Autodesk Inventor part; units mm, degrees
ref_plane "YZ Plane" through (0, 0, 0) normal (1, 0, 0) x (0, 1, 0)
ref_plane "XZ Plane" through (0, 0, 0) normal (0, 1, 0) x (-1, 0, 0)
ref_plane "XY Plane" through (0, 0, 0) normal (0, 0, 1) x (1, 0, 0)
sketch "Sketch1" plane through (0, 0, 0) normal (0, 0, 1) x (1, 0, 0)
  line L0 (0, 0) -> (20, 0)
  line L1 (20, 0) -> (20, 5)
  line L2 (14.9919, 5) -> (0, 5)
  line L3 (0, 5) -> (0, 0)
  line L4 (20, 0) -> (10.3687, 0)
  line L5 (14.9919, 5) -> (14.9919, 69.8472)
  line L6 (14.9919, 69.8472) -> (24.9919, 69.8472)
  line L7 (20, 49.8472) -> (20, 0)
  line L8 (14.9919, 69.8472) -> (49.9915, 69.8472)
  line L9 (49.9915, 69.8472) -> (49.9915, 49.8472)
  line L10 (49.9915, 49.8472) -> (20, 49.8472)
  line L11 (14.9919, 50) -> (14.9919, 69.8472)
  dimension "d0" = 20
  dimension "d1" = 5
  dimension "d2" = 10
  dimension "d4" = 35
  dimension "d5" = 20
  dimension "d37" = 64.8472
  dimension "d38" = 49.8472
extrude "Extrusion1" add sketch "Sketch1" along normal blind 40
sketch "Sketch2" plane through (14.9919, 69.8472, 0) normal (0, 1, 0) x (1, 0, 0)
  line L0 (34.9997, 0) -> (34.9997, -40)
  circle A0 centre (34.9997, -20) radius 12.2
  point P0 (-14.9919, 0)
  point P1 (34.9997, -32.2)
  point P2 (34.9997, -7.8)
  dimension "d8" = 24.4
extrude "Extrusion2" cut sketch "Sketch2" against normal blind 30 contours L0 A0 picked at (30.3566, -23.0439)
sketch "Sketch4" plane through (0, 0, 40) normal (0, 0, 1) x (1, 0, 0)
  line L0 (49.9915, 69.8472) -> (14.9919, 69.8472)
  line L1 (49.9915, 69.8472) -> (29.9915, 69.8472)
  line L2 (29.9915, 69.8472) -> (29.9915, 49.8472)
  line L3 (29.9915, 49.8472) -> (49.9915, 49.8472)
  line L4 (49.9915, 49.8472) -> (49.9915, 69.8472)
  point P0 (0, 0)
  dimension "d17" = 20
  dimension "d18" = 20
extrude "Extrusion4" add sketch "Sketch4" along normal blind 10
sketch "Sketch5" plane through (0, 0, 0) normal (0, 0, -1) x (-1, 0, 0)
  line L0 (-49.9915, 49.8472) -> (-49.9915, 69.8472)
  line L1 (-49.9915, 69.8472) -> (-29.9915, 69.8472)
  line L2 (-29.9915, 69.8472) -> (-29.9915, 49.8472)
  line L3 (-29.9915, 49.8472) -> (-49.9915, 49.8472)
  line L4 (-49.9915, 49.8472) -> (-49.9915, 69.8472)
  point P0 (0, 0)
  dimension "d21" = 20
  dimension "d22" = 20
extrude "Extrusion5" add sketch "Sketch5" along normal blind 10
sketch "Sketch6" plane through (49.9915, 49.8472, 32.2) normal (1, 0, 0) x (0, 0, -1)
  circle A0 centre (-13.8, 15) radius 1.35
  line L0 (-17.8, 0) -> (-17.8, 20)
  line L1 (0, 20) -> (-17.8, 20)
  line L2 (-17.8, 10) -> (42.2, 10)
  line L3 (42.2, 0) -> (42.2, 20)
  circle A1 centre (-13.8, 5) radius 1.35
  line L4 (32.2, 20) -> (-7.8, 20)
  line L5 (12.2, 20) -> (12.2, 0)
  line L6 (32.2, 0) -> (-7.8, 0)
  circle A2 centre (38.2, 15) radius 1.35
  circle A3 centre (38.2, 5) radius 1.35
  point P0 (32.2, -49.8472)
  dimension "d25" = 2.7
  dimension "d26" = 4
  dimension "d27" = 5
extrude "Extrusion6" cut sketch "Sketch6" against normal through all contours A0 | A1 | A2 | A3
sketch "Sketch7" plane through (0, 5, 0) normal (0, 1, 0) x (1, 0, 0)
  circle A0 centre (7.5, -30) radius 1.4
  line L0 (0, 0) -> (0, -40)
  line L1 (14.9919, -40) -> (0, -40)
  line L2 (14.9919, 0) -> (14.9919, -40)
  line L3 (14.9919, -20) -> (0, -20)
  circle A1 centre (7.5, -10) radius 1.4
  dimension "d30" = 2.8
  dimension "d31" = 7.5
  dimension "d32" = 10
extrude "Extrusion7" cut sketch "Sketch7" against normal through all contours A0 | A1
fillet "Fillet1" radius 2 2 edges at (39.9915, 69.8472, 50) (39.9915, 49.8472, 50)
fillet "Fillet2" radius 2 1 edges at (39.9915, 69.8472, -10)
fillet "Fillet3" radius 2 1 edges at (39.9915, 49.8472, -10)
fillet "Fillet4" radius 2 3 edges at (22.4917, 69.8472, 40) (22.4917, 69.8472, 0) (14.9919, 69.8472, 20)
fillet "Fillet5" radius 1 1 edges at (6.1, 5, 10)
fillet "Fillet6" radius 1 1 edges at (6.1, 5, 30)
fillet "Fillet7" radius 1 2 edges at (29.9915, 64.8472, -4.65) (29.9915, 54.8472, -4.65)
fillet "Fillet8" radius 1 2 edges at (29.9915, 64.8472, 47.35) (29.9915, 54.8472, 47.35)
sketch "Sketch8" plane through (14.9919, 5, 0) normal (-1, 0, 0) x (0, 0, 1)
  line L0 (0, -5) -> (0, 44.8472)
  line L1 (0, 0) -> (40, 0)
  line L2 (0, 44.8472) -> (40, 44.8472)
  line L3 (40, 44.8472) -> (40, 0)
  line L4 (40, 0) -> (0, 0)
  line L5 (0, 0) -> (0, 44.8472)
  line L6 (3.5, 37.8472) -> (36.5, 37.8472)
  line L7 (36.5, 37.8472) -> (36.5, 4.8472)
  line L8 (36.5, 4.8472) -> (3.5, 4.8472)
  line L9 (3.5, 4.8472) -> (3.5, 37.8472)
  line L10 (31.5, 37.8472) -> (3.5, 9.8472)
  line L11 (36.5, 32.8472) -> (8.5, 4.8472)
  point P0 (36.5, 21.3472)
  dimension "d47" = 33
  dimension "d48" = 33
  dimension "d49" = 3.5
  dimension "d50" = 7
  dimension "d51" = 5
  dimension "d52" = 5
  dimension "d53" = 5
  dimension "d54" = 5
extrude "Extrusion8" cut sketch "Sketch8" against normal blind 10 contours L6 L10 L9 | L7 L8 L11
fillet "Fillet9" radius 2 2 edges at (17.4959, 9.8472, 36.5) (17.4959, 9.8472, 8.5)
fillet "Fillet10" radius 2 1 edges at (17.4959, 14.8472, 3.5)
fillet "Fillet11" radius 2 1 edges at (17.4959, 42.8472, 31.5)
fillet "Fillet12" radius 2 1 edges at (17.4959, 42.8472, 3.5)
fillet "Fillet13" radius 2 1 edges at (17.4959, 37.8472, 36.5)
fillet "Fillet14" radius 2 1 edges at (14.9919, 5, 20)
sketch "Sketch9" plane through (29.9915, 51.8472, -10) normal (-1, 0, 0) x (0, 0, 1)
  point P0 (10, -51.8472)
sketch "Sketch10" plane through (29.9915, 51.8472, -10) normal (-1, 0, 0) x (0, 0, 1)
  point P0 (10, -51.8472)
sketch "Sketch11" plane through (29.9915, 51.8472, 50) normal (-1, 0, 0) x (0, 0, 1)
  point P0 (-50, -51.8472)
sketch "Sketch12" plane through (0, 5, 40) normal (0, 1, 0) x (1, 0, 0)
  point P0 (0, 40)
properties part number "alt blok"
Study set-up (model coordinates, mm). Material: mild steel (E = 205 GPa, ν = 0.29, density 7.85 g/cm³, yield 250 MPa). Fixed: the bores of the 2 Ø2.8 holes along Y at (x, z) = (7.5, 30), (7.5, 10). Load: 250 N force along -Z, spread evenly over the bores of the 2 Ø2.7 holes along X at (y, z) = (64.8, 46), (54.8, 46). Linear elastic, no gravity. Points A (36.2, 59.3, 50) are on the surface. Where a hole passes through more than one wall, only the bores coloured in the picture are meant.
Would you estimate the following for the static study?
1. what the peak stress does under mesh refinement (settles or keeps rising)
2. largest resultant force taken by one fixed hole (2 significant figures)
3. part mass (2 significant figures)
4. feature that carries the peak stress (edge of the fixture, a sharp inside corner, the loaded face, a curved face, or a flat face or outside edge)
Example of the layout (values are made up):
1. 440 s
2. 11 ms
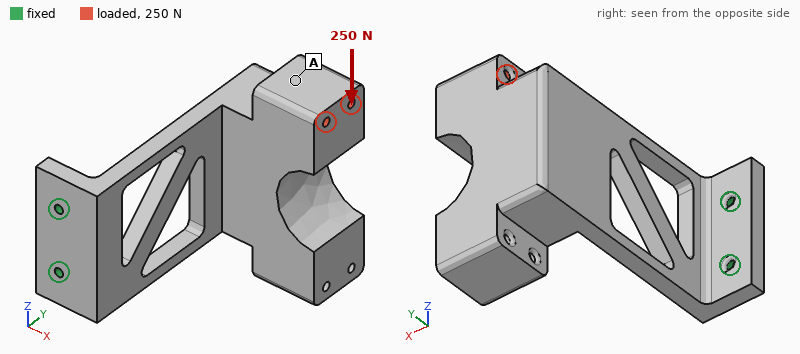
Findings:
1. keeps rising
2. 710 N
3. 310 g
4. edge of the fixture
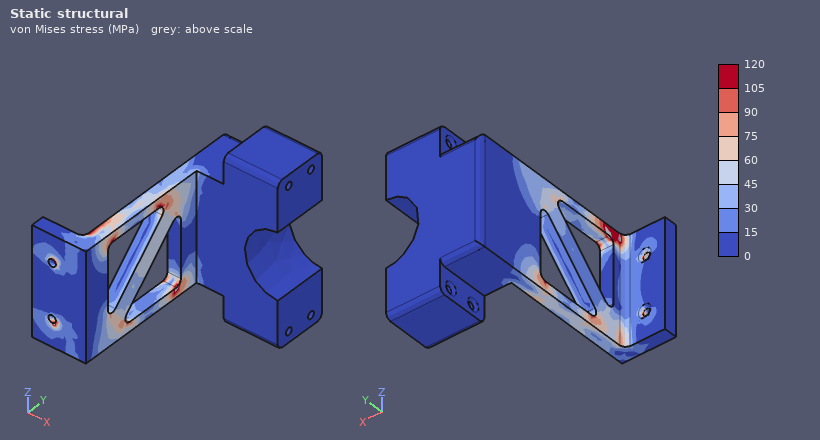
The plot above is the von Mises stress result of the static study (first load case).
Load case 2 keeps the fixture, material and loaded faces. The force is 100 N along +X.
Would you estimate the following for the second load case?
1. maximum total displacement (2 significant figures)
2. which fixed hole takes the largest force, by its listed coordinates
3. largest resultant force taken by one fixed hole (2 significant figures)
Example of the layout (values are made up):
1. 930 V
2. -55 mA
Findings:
1. 0.40 mm
2. (7.5, 30)
3. 170 N
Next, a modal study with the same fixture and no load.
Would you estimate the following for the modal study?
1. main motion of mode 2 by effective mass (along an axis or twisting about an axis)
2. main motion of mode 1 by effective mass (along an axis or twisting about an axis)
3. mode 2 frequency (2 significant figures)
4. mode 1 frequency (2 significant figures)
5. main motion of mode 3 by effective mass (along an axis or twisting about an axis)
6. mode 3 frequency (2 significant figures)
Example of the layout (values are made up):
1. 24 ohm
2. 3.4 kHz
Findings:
1. along Z
2. along X
3. 500 Hz
4. 190 Hz
5. along Z
6. 1000 Hz
